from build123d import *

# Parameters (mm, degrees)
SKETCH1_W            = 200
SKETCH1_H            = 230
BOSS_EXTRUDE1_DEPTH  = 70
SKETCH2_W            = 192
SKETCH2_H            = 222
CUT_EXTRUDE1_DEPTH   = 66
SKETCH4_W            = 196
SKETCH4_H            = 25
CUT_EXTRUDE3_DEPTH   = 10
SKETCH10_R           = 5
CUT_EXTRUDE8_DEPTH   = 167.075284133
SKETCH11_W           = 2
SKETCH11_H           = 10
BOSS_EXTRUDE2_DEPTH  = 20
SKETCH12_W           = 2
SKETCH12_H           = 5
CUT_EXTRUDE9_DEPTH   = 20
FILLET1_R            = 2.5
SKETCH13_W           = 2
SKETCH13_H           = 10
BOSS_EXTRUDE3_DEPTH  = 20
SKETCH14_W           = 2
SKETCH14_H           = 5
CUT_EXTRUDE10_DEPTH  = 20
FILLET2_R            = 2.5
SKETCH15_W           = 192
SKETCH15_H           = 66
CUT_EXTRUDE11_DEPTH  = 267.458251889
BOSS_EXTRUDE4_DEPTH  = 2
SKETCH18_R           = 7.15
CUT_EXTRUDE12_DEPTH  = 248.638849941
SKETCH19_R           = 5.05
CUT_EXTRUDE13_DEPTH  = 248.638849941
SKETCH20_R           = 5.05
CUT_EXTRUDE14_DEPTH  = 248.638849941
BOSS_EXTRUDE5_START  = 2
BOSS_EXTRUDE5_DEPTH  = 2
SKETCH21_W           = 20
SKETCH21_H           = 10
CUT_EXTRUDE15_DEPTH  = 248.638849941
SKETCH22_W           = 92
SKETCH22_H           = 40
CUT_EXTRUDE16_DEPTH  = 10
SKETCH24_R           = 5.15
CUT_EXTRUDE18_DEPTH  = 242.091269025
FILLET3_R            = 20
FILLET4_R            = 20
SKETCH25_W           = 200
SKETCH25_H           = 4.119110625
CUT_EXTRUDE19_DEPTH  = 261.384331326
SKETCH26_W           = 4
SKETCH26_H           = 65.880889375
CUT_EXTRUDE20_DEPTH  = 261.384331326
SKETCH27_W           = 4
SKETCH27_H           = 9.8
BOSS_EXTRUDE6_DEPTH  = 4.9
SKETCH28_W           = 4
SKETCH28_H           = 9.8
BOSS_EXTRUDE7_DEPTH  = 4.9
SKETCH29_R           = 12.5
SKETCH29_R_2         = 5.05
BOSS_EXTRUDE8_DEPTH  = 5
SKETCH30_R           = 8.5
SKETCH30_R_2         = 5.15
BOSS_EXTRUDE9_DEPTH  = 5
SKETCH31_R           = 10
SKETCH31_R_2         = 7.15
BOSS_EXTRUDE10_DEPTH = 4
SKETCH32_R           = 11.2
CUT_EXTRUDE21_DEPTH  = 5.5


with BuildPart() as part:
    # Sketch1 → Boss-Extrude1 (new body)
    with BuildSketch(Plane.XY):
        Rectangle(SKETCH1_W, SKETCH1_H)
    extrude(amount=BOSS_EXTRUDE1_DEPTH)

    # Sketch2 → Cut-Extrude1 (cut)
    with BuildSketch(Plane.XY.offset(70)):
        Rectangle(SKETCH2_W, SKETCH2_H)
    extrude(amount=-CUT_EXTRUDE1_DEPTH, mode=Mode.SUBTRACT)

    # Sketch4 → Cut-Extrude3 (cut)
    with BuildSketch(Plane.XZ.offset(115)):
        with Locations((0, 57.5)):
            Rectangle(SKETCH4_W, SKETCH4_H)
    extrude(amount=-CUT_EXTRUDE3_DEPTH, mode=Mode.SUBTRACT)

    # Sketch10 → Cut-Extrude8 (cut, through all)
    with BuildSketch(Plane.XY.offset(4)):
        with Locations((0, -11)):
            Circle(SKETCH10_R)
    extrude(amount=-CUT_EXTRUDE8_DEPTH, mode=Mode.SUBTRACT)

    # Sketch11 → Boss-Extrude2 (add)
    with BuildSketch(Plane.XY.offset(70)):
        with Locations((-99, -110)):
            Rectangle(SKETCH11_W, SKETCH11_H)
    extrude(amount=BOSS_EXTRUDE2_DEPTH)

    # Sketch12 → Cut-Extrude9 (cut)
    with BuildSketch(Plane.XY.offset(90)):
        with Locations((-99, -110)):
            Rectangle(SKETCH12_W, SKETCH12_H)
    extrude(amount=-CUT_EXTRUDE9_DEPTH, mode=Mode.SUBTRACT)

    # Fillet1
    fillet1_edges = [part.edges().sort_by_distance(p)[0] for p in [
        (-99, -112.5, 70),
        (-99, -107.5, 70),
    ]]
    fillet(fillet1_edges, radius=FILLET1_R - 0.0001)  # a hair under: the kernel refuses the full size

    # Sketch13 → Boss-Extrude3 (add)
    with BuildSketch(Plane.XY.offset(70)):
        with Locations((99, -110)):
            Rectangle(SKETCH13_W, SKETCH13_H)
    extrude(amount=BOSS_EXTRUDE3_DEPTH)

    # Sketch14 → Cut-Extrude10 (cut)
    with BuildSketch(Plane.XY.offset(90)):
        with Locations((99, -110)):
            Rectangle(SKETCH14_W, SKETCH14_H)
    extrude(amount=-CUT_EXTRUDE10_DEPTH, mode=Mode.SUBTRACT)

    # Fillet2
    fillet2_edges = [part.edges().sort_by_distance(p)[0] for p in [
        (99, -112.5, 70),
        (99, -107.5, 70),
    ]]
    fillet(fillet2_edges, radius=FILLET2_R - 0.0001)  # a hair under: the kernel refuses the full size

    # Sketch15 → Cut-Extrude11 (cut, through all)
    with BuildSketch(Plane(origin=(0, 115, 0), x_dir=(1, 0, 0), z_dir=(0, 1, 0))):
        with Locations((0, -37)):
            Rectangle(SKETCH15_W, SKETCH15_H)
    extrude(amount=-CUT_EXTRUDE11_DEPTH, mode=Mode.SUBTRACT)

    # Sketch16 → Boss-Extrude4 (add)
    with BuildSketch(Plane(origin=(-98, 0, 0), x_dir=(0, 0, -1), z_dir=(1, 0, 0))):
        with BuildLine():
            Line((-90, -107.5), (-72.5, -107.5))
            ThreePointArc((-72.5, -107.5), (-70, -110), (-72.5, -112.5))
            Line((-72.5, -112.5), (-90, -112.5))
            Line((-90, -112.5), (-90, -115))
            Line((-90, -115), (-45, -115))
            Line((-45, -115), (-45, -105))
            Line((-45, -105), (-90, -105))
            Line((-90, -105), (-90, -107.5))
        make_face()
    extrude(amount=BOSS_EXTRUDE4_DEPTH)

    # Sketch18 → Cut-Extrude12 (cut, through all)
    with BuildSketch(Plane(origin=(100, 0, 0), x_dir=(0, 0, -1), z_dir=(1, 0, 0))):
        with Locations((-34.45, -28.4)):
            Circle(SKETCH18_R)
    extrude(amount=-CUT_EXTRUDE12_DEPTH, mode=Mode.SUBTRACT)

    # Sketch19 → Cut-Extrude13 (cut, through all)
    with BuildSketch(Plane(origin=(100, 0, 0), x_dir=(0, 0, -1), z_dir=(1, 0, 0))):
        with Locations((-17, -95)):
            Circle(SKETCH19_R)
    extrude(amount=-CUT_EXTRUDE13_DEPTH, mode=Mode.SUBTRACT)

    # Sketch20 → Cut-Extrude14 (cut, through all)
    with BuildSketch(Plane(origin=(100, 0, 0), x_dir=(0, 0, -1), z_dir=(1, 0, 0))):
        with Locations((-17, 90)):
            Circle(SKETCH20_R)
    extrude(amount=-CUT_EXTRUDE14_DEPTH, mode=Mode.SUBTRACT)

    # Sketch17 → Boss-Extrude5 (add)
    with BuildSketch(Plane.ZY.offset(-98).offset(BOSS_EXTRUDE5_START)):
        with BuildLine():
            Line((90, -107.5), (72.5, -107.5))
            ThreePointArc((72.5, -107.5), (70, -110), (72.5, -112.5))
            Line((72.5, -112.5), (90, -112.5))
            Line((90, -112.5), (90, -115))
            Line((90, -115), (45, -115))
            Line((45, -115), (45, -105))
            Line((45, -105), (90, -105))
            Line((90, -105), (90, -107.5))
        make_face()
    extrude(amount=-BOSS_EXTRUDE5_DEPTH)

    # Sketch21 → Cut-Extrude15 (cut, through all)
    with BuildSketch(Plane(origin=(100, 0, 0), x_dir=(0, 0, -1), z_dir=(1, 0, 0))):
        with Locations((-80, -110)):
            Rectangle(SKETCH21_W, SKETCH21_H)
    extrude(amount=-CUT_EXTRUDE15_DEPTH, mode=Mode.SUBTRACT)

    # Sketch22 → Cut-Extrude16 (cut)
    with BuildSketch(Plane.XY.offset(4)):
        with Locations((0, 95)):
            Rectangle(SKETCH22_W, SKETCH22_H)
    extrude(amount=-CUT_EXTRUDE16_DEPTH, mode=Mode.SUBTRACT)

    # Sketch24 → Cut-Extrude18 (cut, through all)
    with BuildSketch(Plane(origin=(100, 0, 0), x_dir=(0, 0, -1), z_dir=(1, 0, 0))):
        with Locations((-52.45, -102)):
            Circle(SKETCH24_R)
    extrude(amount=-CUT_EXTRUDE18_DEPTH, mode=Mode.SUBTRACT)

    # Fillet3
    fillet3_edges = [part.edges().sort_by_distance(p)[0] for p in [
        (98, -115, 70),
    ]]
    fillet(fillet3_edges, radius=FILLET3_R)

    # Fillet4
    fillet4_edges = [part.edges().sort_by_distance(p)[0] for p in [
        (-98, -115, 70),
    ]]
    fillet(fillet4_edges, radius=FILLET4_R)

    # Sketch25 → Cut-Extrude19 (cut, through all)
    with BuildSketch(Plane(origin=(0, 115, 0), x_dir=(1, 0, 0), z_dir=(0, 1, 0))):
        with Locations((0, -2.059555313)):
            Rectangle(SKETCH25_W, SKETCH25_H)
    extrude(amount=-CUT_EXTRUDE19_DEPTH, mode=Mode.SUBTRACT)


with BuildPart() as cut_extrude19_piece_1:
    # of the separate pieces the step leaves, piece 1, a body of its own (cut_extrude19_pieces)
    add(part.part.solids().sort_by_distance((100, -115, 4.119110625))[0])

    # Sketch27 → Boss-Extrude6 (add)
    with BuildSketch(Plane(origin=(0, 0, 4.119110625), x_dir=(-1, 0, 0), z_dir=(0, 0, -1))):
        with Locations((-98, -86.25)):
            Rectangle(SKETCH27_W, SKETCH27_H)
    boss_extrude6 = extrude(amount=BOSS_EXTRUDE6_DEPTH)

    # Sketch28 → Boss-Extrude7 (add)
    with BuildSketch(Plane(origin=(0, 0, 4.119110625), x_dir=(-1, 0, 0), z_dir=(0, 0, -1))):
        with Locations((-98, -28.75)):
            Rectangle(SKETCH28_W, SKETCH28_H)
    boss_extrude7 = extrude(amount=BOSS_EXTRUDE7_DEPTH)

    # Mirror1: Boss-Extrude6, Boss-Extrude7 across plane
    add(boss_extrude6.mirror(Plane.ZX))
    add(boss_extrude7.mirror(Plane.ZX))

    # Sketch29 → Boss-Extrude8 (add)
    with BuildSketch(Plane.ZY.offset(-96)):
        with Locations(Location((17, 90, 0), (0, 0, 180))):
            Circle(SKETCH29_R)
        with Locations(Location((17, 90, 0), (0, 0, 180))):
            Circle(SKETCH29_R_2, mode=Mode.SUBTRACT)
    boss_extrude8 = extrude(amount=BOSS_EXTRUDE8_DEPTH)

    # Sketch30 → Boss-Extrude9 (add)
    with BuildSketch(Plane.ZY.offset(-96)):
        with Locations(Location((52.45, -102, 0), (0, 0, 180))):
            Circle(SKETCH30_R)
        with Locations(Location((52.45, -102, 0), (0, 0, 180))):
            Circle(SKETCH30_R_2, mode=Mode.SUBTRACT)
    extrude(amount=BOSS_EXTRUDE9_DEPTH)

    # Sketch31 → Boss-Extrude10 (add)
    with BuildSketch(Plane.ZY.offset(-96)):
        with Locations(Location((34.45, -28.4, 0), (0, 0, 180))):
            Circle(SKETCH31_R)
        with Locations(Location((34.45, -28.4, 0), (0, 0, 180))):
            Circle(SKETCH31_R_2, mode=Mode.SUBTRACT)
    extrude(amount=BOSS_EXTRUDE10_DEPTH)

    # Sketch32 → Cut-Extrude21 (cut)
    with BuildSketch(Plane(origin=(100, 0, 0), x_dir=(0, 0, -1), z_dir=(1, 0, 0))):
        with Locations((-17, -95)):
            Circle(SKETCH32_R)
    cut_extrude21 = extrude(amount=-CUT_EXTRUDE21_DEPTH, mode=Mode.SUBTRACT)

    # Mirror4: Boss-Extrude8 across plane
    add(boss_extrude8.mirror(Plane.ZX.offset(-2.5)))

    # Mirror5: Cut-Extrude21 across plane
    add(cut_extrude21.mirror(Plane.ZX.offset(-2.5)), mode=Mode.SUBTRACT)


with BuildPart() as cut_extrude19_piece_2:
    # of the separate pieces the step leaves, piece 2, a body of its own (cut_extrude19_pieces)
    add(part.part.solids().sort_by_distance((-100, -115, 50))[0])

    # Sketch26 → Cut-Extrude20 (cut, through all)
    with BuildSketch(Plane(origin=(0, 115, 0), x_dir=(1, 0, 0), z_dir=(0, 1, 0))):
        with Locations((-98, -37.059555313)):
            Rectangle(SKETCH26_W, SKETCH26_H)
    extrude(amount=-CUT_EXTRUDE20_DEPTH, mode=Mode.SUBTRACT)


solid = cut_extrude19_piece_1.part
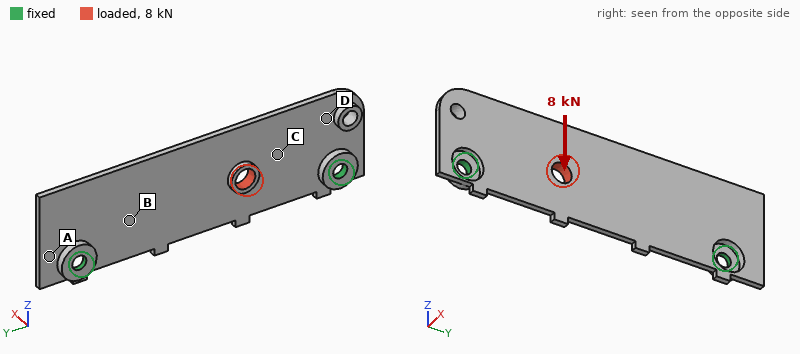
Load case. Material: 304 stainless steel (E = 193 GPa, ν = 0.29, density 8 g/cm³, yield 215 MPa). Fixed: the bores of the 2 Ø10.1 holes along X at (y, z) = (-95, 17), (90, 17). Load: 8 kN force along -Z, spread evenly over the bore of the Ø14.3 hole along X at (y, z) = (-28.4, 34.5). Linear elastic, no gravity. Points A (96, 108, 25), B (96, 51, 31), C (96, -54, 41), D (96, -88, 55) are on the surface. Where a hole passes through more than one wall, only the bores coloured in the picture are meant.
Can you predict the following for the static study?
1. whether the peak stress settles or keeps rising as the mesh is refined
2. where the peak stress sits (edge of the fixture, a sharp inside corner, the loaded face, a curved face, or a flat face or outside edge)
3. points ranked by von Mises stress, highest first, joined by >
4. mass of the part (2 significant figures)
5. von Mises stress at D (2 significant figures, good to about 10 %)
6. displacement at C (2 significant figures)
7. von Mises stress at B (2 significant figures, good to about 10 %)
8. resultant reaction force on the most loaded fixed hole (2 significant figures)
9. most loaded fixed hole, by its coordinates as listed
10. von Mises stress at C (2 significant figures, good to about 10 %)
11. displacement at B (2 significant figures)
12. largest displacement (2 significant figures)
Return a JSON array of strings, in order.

["keeps rising", "edge of the fixture", "C > B > D > A", "500 g", "40 MPa", "0.047 mm", "55 MPa", "5.7 kN", "(-95, 17)", "93 MPa", "0.038 mm", "0.18 mm"]
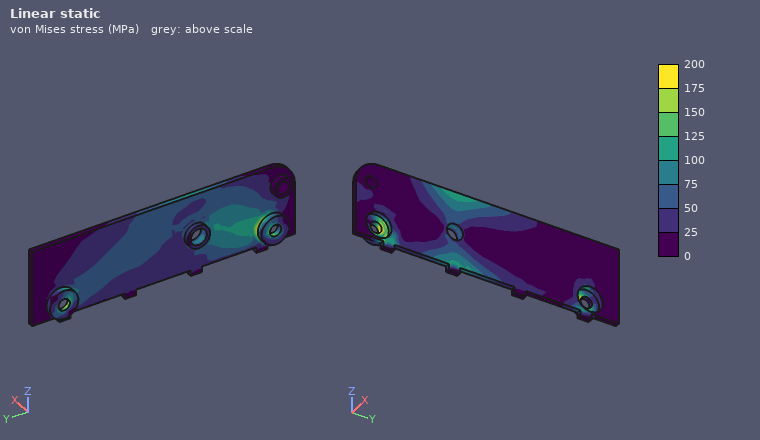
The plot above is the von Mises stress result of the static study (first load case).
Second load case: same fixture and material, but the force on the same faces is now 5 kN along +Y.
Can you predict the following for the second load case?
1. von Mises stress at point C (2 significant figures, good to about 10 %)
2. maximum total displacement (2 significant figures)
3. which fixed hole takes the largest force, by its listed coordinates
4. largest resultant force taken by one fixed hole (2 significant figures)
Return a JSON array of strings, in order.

["35 MPa", "70 µm", "(-95, 17)", "3.2 kN"]
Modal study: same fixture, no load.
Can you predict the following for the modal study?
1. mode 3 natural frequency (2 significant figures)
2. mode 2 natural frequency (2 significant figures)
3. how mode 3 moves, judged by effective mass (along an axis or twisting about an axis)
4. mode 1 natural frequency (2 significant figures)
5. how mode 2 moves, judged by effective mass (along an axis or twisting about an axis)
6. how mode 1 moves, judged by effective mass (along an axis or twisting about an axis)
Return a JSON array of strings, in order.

["1200 Hz", "940 Hz", "twisting about Z", "520 Hz", "twisting about Y", "along X"]
